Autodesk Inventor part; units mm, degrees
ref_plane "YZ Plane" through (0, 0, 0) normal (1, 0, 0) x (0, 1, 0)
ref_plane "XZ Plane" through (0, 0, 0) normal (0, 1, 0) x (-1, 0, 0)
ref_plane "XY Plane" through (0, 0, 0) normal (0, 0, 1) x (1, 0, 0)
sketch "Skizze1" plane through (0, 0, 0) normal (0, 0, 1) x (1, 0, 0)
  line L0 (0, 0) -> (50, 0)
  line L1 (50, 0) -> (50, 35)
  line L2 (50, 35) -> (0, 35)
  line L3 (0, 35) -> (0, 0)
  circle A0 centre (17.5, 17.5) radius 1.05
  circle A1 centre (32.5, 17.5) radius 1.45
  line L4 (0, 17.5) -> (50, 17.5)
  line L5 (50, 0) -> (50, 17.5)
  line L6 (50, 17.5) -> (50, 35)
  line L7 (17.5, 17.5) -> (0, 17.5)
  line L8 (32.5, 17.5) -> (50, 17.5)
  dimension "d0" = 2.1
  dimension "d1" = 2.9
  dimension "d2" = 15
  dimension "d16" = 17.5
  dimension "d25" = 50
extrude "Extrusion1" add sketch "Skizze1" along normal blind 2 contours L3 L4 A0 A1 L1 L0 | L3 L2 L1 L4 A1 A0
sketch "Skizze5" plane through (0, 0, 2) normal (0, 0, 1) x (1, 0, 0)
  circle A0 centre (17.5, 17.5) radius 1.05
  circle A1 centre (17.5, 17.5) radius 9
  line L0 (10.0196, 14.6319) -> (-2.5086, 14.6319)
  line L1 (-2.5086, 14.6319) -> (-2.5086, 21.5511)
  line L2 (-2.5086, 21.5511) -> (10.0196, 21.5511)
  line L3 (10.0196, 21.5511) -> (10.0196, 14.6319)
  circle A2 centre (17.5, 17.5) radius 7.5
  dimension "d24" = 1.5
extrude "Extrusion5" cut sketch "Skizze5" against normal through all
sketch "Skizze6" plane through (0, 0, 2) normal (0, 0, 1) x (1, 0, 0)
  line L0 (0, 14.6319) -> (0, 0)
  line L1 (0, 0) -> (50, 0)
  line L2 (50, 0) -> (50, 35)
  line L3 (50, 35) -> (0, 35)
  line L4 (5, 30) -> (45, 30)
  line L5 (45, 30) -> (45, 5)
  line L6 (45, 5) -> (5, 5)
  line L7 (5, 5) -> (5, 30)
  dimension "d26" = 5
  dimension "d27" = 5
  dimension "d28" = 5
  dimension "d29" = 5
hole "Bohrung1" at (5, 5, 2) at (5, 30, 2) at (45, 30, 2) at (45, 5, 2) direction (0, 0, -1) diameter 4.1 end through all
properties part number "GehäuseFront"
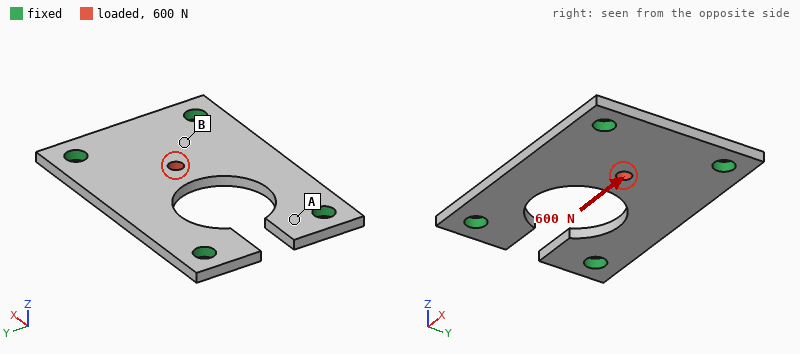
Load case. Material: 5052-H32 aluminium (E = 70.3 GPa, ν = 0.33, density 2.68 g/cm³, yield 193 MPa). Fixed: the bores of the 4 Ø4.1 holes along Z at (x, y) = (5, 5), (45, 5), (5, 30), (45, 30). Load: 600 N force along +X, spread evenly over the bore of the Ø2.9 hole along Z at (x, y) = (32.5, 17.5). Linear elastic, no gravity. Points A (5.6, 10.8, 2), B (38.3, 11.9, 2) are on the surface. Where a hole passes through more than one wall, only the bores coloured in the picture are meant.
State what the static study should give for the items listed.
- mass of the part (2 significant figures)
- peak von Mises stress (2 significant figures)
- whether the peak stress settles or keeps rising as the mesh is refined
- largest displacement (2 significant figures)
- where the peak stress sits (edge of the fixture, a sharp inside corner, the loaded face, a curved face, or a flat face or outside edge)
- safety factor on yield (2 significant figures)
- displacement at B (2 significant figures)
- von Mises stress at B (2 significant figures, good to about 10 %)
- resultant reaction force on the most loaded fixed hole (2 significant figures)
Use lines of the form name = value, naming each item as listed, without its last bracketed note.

mass of the part = 7.4 g
peak von Mises stress = 61 MPa
whether the peak stress settles or keeps rising as the mesh is refined = settles
largest displacement = 5.6 µm
where the peak stress sits = the loaded face
safety factor on yield = 3.2
displacement at B = 2.3 µm
von Mises stress at B = 15 MPa
resultant reaction force on the most loaded fixed hole = 270 N
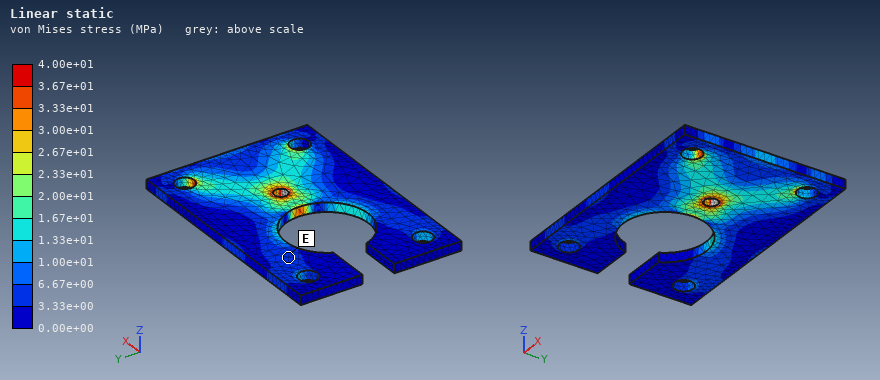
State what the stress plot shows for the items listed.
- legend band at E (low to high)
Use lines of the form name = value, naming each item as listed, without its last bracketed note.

legend band at E = 3.33e+00 to 6.67e+00 MPa
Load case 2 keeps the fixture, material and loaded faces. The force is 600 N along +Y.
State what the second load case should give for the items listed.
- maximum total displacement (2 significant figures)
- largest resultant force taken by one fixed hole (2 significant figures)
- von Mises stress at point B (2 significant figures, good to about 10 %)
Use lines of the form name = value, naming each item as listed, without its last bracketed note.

maximum total displacement = 6.1 µm
largest resultant force taken by one fixed hole = 310 N
von Mises stress at point B = 17 MPa
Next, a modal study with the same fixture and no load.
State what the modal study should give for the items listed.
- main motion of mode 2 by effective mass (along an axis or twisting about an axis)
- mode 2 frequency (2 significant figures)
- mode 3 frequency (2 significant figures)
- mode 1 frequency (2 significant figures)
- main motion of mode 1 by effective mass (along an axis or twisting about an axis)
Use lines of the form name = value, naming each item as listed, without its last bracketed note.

main motion of mode 2 by effective mass = twisting about X
mode 2 frequency = 8600 Hz
mode 3 frequency = 13 kHz
mode 1 frequency = 6900 Hz
main motion of mode 1 by effective mass = along Z
